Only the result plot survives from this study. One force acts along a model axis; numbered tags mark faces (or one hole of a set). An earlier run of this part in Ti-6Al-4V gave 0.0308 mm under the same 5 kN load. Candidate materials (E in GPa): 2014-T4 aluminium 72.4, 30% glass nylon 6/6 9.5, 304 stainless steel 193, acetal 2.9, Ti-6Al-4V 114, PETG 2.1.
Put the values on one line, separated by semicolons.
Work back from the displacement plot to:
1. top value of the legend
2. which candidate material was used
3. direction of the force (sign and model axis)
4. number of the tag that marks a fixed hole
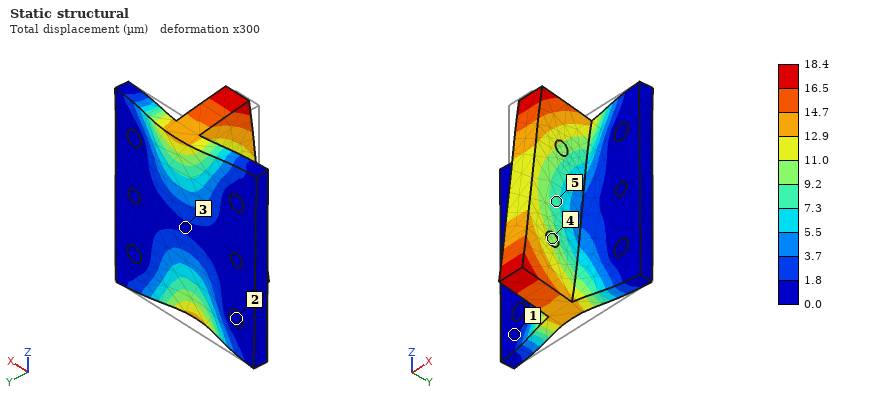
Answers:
18.4 µm; 304 stainless steel; +Z; 2
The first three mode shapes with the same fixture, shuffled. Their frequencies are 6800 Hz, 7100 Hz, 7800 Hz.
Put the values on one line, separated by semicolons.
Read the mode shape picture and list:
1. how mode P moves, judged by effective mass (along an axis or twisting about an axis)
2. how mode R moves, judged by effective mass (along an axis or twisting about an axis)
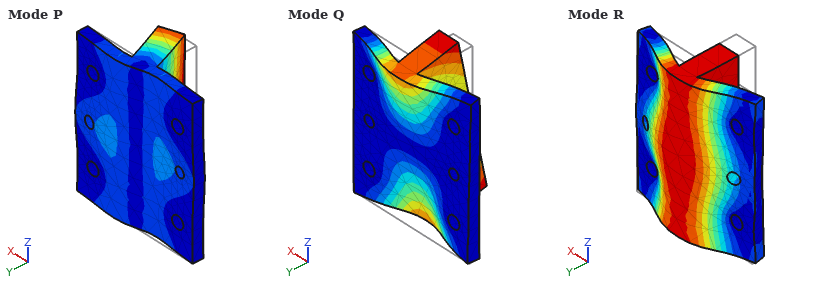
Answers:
along X; along Y
